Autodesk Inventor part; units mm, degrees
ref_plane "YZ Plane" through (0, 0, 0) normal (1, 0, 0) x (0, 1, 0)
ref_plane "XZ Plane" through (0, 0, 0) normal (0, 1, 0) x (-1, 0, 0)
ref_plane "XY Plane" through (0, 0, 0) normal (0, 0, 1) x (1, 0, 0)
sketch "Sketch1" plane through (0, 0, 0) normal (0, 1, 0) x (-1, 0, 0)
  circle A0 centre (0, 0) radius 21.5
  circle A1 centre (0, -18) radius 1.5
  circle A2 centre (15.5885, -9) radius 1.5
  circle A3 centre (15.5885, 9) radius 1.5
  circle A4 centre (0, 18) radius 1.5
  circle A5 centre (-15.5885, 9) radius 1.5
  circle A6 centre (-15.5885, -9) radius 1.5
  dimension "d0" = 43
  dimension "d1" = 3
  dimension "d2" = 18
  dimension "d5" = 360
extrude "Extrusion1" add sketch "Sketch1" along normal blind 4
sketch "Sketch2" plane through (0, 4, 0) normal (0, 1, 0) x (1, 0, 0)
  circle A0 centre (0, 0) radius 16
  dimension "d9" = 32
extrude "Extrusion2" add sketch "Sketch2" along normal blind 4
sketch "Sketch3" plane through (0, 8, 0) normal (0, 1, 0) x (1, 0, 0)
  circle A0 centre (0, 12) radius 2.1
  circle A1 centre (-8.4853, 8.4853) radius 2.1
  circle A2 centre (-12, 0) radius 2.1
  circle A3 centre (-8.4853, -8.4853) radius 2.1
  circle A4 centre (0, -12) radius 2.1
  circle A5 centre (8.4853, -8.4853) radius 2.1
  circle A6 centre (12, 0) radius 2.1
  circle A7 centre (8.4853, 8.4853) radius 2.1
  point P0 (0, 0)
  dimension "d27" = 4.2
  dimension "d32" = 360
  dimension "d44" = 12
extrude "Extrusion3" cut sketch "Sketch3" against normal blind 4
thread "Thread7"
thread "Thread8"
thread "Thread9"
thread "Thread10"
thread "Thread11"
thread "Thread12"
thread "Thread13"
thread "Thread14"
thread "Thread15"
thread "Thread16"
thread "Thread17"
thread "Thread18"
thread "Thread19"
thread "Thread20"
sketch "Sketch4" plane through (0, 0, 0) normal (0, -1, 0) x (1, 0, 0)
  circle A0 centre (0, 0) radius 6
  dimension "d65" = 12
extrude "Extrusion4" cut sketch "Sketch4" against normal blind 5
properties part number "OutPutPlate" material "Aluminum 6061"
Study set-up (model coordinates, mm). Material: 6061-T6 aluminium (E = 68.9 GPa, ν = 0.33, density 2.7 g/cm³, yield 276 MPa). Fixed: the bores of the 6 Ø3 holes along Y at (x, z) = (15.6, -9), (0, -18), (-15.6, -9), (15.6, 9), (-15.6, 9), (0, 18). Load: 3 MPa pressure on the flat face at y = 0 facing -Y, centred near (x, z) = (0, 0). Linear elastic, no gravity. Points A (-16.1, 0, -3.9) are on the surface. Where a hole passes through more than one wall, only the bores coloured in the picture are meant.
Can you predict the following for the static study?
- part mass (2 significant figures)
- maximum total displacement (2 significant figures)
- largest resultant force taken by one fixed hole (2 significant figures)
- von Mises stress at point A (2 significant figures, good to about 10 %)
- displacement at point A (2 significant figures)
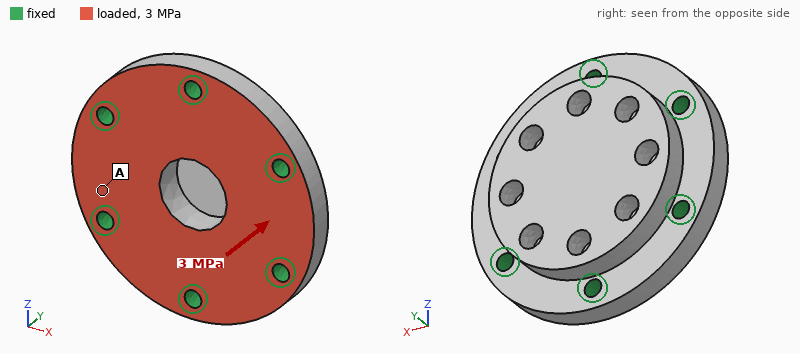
21 g
4.8 µm
660 N
11 MPa
2.3 µm
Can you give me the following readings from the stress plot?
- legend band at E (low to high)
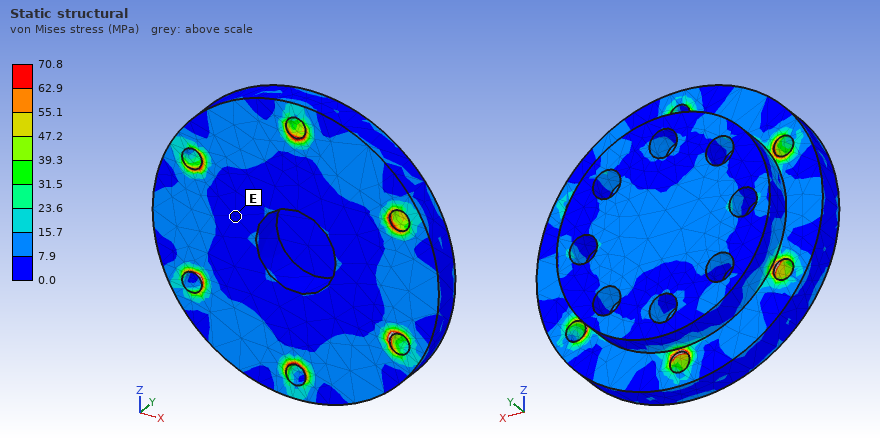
0.0 to 7.9 MPa
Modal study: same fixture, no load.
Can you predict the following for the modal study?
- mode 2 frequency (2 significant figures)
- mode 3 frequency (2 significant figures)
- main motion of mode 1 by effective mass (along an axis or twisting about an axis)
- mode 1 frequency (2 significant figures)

46 kHz
46 kHz
along Y
31 kHz
